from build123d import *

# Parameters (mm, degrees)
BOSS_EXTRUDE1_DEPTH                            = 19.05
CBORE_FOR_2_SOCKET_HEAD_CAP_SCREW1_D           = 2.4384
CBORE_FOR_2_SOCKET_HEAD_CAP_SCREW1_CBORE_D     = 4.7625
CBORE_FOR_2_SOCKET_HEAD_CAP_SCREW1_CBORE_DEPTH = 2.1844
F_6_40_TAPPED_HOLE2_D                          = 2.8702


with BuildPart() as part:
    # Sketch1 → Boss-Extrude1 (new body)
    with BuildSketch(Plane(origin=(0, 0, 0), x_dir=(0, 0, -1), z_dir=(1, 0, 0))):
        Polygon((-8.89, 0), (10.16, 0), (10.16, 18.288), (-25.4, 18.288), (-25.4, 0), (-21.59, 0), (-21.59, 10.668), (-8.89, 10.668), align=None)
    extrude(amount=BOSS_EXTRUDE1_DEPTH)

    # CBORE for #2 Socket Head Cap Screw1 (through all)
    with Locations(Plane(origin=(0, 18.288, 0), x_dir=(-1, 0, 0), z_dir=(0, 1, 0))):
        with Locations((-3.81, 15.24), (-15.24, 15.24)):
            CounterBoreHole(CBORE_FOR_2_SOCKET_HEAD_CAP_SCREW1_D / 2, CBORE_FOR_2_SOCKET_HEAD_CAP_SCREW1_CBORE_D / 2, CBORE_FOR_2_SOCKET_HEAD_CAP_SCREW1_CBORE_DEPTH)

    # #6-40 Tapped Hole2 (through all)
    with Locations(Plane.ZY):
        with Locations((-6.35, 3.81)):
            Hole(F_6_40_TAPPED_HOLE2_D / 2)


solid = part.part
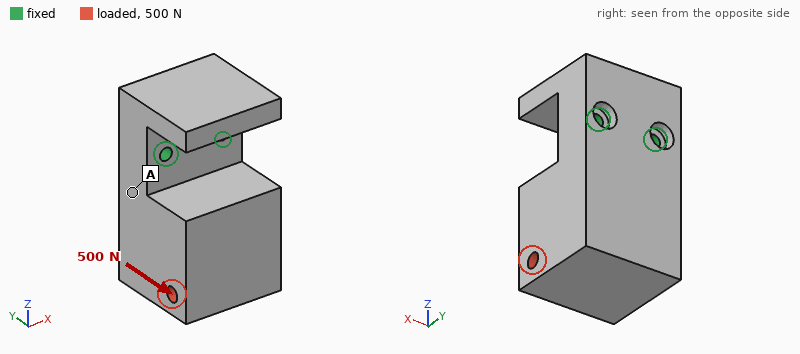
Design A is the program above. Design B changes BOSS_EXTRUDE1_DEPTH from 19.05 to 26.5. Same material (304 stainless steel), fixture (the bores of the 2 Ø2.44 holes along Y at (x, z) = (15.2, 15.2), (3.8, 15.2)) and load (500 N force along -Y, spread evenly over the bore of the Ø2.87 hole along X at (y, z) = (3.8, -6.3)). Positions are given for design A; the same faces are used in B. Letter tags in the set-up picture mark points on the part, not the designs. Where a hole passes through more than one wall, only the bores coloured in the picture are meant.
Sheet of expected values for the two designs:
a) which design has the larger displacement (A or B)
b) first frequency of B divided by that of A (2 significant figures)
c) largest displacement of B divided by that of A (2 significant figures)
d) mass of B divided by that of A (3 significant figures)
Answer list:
A
0.90
0.89
1.40
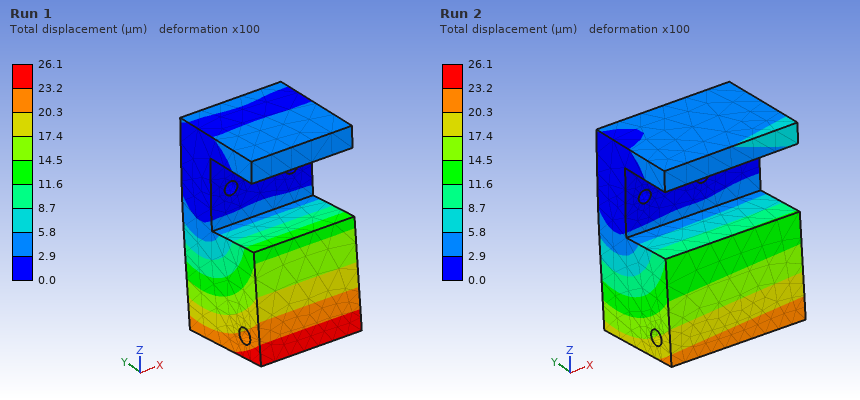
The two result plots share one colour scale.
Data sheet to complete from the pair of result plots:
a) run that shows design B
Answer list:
Run 2
